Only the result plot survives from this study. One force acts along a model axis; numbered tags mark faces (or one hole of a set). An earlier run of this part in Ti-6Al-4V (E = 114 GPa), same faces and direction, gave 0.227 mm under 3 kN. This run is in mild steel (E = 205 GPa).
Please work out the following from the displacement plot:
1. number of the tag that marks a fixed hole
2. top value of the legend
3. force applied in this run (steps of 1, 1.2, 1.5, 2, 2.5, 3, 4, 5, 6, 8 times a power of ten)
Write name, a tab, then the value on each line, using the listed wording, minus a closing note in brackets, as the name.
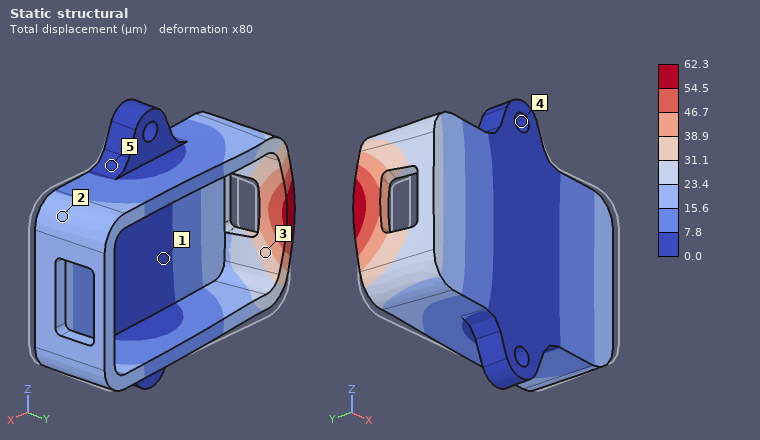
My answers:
number of the tag that marks a fixed hole	4
top value of the legend	62.3 µm
force applied in this run	1.5 kN
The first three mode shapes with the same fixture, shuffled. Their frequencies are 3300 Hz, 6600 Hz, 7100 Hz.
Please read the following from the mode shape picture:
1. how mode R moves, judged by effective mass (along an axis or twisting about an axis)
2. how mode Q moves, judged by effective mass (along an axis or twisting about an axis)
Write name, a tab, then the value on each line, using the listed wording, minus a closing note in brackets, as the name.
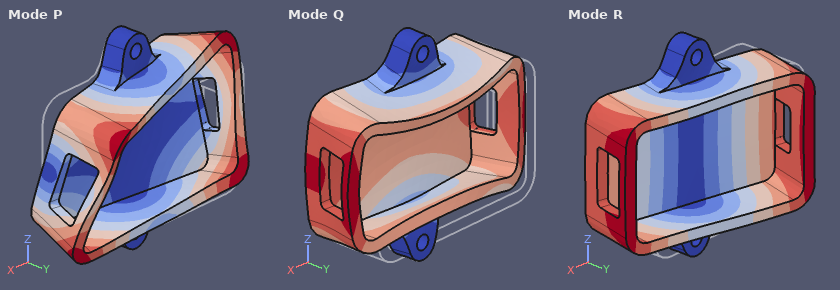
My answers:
how mode R moves, judged by effective mass	twisting about Z
how mode Q moves, judged by effective mass	along Y
